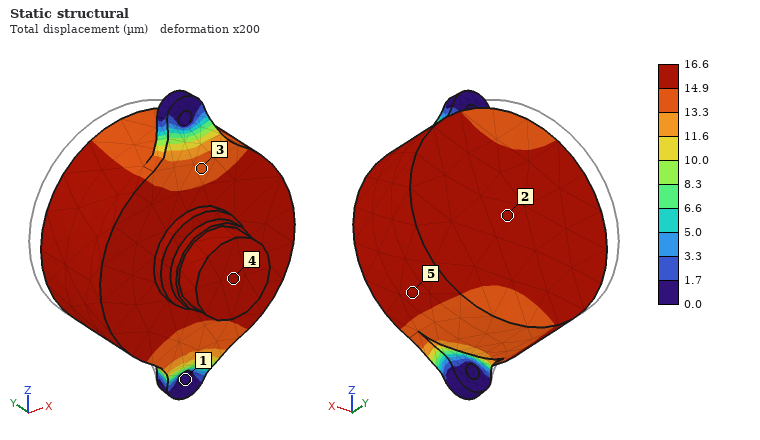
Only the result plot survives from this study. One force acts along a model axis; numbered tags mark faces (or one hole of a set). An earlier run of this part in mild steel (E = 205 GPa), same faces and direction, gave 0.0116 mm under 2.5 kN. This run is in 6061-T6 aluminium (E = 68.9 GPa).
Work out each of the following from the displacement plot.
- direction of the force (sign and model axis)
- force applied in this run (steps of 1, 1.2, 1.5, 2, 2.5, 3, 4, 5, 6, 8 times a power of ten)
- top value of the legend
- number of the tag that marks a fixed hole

-Y
1.2 kN
16.6 µm
1
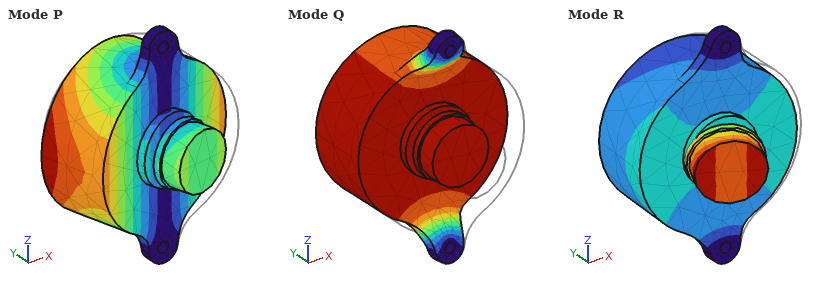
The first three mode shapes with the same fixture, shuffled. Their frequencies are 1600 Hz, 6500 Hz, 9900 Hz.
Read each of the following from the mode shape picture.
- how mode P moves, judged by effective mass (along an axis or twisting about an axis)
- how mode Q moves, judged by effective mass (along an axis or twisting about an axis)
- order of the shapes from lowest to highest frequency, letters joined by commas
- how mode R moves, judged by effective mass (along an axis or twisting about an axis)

along X
along Y
P, Q, R
along X
